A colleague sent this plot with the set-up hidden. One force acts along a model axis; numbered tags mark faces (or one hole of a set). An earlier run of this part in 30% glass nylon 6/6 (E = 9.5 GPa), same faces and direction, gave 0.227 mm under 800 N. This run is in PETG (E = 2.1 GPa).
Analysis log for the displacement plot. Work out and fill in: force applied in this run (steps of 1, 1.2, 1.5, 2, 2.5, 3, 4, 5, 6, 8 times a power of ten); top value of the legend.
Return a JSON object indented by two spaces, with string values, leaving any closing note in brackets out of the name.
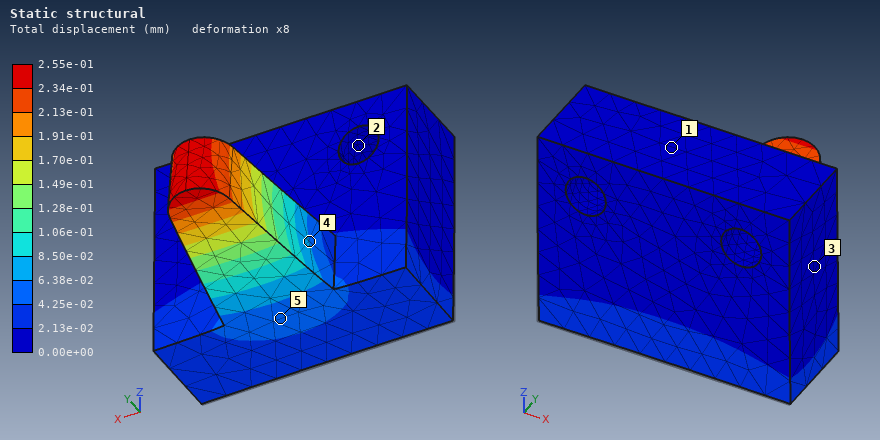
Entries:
{
  "force applied in this run": "200 N",
  "top value of the legend": "2.55e-01 mm"
}
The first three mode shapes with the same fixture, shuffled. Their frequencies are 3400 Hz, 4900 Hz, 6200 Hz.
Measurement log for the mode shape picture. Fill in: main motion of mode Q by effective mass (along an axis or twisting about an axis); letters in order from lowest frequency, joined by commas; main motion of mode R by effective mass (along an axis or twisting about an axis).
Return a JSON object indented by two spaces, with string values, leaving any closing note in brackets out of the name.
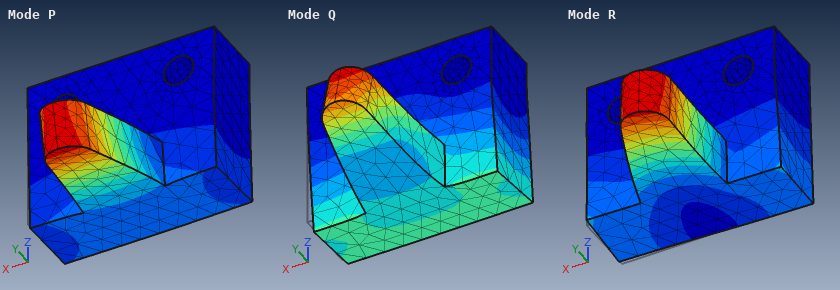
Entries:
{
  "main motion of mode Q by effective mass": "along Y",
  "letters in order from lowest frequency, joined by commas": "P, R, Q",
  "main motion of mode R by effective mass": "along X"
}
